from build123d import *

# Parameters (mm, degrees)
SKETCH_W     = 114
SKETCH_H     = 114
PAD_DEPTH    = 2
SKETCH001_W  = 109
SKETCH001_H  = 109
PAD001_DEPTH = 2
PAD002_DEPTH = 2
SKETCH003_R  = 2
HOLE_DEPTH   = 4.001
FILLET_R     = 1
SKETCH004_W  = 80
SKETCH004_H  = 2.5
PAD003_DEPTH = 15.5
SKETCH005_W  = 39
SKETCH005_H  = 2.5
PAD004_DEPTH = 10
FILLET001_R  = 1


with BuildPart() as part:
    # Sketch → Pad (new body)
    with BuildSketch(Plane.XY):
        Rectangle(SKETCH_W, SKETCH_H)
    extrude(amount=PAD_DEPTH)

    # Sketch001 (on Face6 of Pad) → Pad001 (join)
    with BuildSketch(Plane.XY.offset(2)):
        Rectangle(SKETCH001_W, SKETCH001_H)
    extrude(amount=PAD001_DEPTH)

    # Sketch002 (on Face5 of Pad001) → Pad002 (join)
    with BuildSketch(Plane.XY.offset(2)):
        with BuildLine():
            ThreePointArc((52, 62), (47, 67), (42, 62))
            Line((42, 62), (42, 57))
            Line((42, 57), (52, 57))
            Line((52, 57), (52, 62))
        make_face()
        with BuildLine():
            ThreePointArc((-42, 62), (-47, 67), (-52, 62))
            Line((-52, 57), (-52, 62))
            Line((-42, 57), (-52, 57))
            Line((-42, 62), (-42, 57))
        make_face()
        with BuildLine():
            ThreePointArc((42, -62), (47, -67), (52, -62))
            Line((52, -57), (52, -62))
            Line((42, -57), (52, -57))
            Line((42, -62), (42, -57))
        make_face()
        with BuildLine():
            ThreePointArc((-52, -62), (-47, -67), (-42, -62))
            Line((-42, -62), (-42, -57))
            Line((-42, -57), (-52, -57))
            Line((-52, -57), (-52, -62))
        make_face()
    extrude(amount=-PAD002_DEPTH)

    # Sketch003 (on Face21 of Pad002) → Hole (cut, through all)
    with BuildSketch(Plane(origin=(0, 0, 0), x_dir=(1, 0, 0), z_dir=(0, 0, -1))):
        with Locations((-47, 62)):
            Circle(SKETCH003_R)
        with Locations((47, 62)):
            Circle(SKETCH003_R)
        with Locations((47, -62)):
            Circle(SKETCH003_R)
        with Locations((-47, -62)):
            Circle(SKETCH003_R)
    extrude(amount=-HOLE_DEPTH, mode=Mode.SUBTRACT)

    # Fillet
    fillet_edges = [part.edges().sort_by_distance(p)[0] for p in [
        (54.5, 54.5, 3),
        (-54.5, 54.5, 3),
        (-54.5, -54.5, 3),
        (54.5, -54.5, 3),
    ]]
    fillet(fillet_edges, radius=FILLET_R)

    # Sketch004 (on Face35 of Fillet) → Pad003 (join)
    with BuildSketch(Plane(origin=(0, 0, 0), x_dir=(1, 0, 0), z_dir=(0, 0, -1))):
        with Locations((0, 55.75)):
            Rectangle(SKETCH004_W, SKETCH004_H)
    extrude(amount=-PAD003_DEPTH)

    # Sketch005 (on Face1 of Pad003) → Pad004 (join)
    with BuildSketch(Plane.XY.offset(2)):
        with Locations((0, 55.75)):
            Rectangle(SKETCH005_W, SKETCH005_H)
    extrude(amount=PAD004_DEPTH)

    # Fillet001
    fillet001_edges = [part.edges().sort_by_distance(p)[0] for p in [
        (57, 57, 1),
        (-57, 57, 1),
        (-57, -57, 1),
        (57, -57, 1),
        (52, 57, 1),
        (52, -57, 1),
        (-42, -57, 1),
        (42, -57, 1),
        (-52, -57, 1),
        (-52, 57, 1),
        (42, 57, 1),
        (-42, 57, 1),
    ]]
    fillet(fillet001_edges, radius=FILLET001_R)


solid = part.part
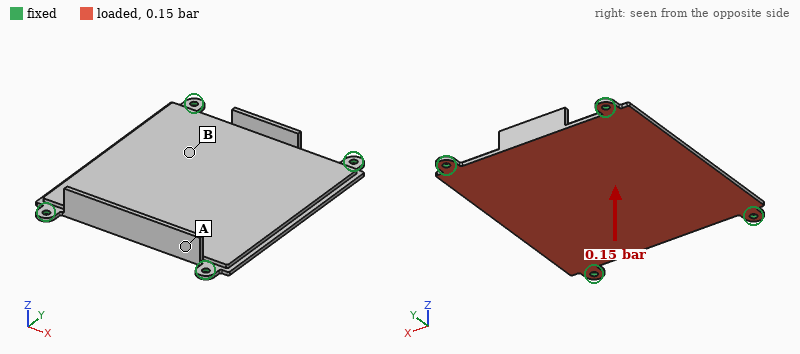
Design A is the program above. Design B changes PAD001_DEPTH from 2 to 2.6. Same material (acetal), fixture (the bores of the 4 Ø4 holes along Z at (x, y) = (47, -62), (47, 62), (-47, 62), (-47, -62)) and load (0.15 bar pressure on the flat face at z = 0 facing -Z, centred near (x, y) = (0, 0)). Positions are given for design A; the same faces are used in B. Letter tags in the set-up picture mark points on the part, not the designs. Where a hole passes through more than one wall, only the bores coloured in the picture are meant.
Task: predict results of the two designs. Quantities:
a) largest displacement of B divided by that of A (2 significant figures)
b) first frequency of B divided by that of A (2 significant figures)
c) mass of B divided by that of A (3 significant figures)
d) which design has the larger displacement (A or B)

0.69
1.1
1.13
A
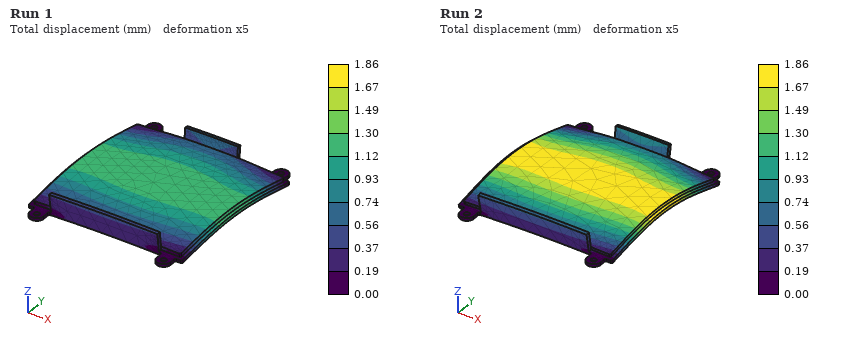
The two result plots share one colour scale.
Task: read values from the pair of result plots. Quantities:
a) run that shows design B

Run 1
